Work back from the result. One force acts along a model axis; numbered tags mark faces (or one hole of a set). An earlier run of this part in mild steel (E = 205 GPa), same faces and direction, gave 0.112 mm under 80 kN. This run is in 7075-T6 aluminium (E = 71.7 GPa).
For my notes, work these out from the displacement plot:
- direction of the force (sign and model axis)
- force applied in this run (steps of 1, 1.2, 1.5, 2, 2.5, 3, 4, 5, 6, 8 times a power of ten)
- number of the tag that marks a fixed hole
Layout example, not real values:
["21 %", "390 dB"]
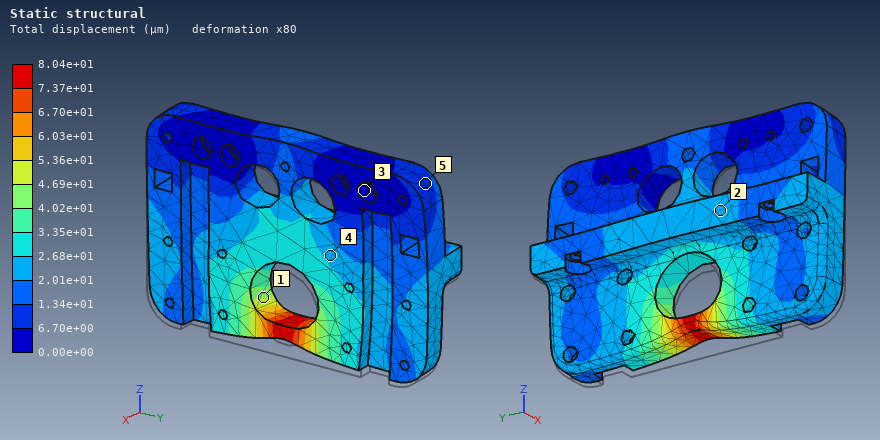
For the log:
["+Z", "20 kN", "3"]
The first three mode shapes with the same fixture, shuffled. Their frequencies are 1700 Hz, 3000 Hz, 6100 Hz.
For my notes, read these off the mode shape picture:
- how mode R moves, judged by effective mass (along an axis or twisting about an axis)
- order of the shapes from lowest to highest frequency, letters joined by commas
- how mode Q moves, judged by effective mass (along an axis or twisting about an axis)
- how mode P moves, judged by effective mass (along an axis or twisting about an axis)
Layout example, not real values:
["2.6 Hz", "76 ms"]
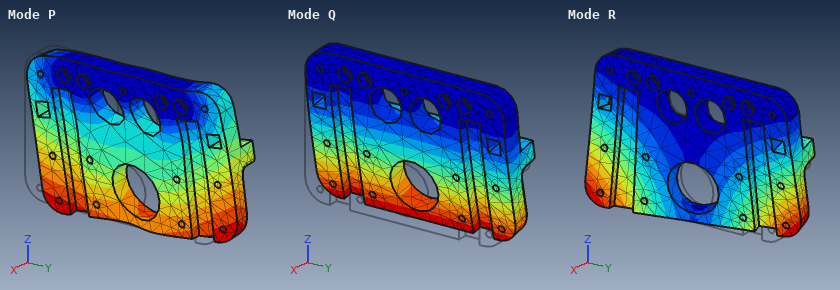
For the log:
["twisting about Z", "Q, R, P", "along X", "along Y"]
